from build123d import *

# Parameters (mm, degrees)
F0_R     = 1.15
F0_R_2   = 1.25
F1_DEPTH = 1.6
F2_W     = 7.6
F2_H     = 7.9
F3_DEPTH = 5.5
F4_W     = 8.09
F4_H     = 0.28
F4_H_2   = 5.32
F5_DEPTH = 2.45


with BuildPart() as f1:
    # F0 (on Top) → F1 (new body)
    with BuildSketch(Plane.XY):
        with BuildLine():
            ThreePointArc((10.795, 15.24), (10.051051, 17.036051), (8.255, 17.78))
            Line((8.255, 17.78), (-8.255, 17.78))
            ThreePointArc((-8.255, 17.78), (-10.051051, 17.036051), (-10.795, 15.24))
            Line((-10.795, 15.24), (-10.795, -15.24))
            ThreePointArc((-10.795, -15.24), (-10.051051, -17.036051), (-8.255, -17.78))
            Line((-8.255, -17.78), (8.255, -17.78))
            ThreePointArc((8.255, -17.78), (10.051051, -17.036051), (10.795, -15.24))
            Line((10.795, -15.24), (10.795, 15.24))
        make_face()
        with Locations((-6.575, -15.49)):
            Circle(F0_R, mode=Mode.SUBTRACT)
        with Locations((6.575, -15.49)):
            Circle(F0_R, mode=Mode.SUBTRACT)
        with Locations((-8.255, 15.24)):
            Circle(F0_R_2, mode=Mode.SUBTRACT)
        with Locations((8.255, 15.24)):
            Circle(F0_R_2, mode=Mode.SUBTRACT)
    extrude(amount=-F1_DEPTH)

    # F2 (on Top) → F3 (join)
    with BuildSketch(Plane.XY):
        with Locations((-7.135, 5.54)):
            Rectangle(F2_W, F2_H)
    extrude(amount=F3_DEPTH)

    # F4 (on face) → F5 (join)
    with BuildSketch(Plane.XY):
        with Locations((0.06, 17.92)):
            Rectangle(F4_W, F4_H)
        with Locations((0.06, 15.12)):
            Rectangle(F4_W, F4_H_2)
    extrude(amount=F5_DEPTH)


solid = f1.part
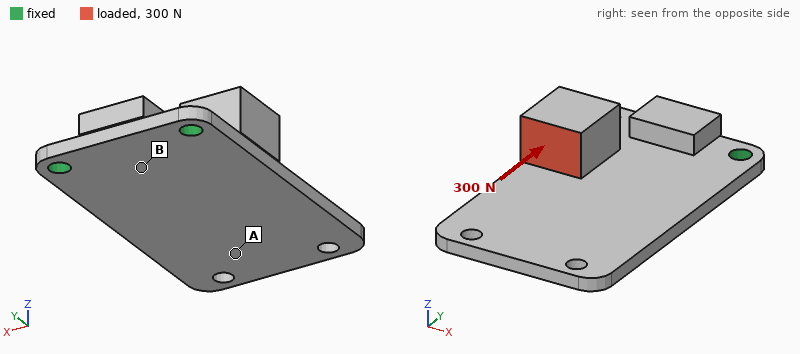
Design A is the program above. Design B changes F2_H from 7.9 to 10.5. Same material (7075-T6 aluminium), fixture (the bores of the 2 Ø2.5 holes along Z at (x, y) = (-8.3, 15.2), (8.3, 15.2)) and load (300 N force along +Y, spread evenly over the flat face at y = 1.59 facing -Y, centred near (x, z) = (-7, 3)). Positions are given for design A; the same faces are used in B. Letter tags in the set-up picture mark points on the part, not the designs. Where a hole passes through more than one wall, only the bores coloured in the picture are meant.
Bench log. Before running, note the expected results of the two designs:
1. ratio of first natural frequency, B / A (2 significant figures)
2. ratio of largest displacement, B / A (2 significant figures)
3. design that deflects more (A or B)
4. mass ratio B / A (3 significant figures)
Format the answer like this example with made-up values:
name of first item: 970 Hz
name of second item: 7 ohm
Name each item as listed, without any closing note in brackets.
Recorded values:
ratio of first natural frequency, B / A: 1.1
ratio of largest displacement, B / A: 0.86
design that deflects more: A
mass ratio B / A: 1.07
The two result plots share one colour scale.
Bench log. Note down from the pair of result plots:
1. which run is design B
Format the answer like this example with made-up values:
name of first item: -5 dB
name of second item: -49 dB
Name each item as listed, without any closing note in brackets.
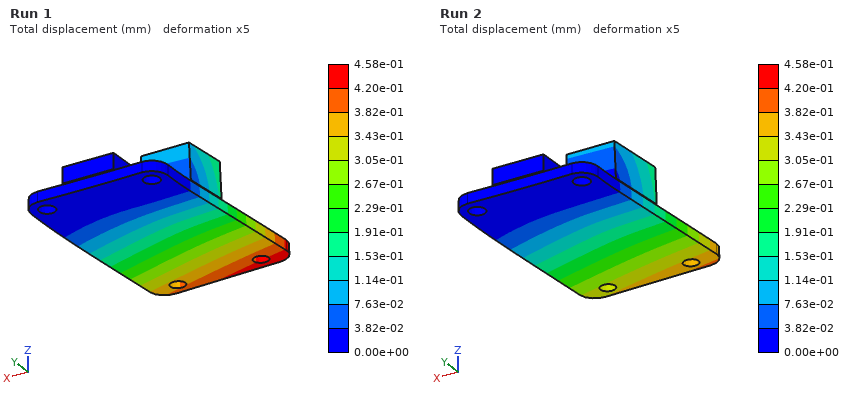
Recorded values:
which run is design B: Run 2
